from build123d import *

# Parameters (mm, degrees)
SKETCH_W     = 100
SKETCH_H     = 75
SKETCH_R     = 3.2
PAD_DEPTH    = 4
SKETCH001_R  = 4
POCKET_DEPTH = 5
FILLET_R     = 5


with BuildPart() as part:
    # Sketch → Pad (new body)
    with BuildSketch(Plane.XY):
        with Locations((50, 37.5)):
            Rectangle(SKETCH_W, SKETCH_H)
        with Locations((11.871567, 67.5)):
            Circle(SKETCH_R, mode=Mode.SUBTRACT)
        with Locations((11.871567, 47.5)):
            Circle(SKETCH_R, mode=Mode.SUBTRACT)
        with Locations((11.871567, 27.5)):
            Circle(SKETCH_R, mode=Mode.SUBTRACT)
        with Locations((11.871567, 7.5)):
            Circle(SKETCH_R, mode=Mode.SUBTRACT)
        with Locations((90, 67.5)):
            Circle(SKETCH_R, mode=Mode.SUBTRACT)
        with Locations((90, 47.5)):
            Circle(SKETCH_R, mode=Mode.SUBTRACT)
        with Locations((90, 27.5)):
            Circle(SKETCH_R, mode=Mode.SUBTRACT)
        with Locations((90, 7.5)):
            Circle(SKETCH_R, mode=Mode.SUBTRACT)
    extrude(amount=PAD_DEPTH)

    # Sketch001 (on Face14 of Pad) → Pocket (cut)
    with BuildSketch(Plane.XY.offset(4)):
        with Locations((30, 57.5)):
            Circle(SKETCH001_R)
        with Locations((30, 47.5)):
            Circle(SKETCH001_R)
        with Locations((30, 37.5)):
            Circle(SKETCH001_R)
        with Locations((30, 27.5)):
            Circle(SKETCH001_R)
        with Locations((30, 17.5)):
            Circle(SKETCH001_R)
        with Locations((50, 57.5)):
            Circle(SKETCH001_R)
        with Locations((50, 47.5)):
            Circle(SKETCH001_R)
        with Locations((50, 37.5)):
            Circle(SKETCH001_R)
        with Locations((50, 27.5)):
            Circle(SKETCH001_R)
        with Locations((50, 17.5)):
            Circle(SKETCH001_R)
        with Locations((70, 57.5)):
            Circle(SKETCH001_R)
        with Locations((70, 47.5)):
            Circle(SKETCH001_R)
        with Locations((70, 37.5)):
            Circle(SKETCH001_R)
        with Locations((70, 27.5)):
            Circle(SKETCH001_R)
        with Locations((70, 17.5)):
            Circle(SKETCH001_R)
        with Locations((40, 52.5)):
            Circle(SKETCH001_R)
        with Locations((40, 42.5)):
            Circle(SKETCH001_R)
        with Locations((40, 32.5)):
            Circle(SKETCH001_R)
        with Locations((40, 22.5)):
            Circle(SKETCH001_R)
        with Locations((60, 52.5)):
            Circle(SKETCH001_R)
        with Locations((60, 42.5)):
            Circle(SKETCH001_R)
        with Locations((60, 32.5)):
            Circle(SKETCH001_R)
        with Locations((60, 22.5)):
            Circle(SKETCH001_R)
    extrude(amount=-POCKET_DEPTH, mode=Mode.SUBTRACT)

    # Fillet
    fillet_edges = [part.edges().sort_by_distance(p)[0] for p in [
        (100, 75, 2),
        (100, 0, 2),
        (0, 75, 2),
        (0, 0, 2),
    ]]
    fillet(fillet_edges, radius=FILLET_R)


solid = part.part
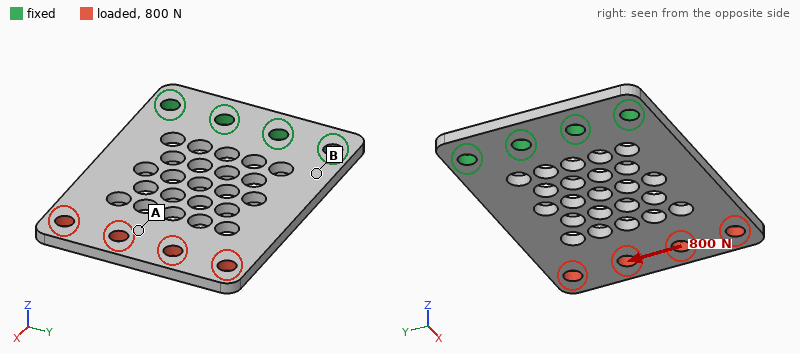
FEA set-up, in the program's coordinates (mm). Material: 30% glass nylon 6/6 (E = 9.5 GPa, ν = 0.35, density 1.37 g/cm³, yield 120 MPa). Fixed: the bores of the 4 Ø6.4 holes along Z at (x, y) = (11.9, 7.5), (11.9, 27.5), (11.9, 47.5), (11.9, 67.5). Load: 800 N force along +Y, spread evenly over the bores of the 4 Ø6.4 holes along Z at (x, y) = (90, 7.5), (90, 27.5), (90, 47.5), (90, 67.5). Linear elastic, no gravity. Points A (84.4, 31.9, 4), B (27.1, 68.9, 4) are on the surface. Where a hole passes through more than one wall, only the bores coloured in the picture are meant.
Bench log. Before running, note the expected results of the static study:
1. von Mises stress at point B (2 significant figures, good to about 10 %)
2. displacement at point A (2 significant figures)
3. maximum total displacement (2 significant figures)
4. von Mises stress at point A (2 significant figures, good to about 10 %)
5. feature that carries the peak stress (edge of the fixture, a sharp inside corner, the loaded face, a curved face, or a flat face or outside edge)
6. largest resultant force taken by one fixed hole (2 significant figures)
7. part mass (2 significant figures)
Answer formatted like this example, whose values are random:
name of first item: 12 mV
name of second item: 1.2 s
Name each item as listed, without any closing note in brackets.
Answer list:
von Mises stress at point B: 18 MPa
displacement at point A: 0.31 mm
maximum total displacement: 0.37 mm
von Mises stress at point A: 7.2 MPa
feature that carries the peak stress: a curved face
largest resultant force taken by one fixed hole: 980 N
part mass: 33 g
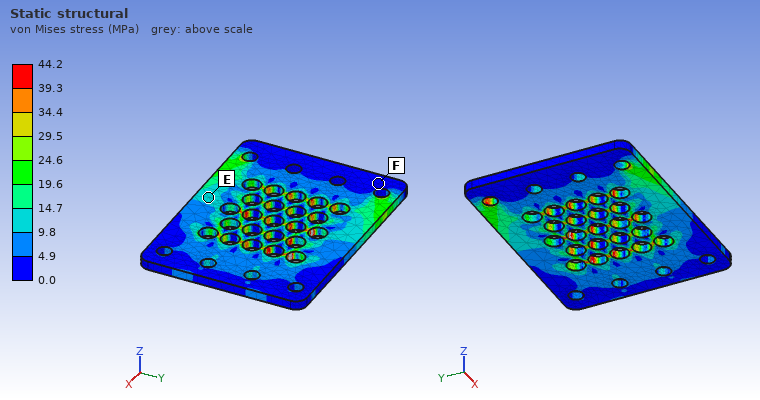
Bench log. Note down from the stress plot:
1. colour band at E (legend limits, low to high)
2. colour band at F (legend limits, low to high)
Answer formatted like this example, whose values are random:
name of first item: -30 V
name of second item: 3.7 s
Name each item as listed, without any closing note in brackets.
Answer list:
colour band at E: 9.8 to 14.7 MPa
colour band at F: 0.0 to 4.9 MPa
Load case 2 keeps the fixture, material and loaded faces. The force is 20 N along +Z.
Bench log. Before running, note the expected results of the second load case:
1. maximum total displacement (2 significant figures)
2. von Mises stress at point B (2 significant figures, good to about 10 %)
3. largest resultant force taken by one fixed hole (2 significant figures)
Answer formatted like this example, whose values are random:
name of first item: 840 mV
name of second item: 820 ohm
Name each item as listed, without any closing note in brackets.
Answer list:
maximum total displacement: 1.4 mm
von Mises stress at point B: 9.6 MPa
largest resultant force taken by one fixed hole: 7.3 N
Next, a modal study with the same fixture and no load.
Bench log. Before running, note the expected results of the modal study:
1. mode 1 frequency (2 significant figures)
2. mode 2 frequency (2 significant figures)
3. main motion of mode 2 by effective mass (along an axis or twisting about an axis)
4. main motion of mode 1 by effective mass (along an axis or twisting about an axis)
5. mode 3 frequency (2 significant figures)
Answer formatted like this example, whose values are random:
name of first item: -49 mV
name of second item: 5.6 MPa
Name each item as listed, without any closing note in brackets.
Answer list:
mode 1 frequency: 200 Hz
mode 2 frequency: 540 Hz
main motion of mode 2 by effective mass: twisting about X
main motion of mode 1 by effective mass: along Z
mode 3 frequency: 1300 Hz
